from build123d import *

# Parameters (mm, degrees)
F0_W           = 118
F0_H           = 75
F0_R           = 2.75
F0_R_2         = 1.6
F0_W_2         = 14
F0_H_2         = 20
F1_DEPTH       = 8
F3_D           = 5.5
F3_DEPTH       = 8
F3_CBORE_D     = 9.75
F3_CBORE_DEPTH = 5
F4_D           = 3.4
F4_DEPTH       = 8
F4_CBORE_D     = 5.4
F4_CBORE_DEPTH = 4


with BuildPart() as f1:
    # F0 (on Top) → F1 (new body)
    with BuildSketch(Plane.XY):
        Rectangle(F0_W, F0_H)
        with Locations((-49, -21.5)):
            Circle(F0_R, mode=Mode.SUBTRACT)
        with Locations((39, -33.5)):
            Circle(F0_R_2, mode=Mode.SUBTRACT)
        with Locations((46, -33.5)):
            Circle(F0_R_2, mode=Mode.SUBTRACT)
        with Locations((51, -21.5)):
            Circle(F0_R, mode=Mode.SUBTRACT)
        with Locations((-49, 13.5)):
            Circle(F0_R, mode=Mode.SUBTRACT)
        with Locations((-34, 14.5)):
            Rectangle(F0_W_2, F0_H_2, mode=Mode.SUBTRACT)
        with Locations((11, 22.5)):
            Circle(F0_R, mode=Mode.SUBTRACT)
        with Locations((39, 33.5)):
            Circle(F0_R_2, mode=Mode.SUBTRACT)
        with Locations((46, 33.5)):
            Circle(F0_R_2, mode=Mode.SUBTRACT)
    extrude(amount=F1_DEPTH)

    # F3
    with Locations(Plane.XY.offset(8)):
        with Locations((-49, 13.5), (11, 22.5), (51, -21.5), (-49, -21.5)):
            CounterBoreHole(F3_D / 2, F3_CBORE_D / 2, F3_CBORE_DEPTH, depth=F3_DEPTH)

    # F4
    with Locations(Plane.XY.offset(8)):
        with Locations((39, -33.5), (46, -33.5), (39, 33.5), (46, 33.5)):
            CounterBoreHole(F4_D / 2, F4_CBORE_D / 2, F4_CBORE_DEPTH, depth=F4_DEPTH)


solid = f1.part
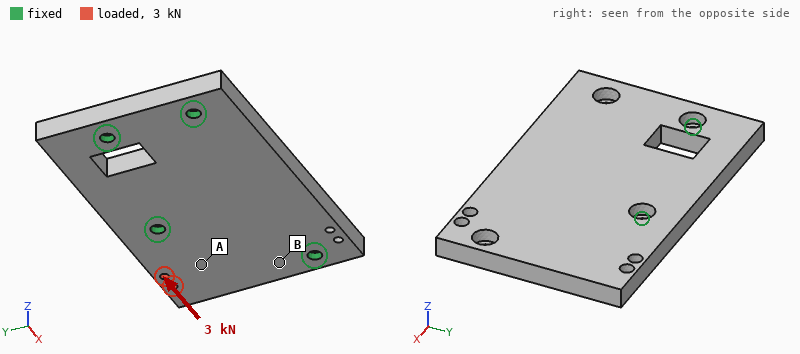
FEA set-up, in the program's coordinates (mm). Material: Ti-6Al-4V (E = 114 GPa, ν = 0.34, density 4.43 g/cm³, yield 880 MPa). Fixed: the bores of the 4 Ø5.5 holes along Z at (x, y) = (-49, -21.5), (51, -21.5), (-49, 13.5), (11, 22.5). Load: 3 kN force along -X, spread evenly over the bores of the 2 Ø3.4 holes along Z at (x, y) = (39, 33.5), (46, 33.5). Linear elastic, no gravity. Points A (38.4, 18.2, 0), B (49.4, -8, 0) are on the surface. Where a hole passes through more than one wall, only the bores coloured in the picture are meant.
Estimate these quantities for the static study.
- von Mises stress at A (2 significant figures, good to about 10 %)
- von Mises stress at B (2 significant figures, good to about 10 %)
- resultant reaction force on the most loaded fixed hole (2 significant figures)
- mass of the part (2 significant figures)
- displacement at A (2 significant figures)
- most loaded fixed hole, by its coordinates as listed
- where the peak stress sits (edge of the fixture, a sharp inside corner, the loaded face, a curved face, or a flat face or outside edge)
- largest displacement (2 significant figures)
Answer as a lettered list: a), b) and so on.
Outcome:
a) 17 MPa
b) 8.7 MPa
c) 2.4 kN
d) 290 g
e) 6.8 µm
f) (11, 22.5)
g) the loaded face
h) 26 µm
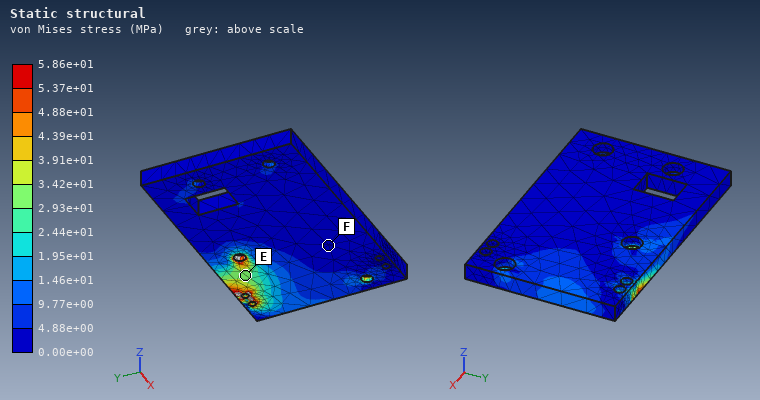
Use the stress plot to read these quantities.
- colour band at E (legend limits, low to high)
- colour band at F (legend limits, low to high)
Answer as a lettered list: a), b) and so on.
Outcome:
a) 2.93e+01 to 3.42e+01 MPa
b) 0.00e+00 to 4.88e+00 MPa
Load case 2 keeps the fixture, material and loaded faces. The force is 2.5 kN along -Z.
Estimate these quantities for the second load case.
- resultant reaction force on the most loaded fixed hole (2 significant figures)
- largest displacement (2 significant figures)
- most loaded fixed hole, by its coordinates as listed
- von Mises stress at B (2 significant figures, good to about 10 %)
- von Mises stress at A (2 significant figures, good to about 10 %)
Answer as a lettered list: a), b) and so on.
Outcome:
a) 4.2 kN
b) 0.33 mm
c) (11, 22.5)
d) 64 MPa
e) 77 MPa
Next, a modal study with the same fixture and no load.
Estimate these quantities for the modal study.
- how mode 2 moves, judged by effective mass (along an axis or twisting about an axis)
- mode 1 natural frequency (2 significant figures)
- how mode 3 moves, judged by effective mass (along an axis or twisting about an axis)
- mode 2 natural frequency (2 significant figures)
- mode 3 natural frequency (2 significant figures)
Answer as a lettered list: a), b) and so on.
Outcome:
a) along Z
b) 3000 Hz
c) along Z
d) 4000 Hz
e) 6100 Hz
